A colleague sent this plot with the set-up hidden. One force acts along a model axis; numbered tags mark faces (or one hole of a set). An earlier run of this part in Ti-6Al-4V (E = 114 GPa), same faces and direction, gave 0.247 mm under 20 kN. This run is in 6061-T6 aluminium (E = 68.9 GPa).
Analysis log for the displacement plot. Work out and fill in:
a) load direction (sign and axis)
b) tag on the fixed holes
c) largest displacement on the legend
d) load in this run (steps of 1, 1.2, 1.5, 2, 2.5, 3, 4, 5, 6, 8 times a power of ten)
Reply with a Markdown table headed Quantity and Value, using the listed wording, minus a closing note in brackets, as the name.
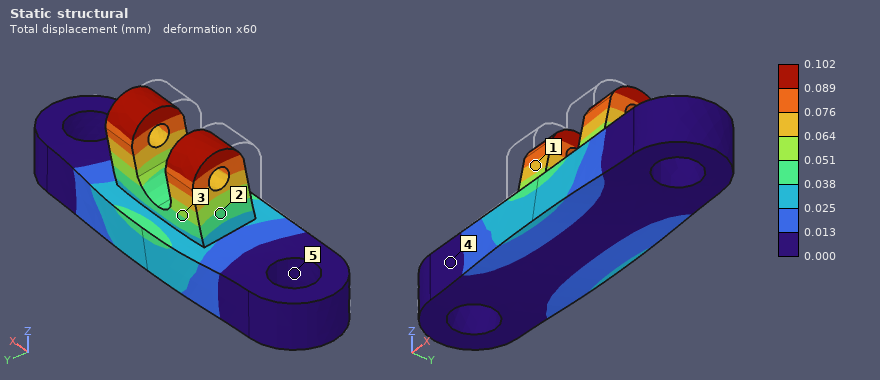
| Quantity | Value |
|---|---|
| load direction | +Y |
| tag on the fixed holes | 5 |
| largest displacement on the legend | 0.102 mm |
| load in this run | 5 kN |
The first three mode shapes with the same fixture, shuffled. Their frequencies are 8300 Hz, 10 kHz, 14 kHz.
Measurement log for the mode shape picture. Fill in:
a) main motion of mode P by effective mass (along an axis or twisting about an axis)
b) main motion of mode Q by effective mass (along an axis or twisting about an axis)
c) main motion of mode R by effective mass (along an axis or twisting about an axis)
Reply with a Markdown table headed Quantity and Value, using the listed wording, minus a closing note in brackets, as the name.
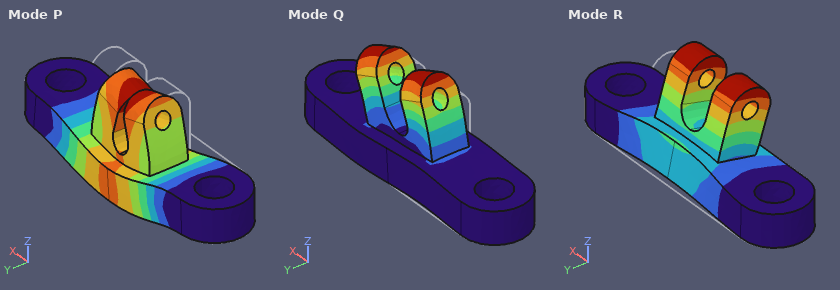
| Quantity | Value |
|---|---|
| main motion of mode P by effective mass | along Z |
| main motion of mode Q by effective mass | along X |
| main motion of mode R by effective mass | along Y |
